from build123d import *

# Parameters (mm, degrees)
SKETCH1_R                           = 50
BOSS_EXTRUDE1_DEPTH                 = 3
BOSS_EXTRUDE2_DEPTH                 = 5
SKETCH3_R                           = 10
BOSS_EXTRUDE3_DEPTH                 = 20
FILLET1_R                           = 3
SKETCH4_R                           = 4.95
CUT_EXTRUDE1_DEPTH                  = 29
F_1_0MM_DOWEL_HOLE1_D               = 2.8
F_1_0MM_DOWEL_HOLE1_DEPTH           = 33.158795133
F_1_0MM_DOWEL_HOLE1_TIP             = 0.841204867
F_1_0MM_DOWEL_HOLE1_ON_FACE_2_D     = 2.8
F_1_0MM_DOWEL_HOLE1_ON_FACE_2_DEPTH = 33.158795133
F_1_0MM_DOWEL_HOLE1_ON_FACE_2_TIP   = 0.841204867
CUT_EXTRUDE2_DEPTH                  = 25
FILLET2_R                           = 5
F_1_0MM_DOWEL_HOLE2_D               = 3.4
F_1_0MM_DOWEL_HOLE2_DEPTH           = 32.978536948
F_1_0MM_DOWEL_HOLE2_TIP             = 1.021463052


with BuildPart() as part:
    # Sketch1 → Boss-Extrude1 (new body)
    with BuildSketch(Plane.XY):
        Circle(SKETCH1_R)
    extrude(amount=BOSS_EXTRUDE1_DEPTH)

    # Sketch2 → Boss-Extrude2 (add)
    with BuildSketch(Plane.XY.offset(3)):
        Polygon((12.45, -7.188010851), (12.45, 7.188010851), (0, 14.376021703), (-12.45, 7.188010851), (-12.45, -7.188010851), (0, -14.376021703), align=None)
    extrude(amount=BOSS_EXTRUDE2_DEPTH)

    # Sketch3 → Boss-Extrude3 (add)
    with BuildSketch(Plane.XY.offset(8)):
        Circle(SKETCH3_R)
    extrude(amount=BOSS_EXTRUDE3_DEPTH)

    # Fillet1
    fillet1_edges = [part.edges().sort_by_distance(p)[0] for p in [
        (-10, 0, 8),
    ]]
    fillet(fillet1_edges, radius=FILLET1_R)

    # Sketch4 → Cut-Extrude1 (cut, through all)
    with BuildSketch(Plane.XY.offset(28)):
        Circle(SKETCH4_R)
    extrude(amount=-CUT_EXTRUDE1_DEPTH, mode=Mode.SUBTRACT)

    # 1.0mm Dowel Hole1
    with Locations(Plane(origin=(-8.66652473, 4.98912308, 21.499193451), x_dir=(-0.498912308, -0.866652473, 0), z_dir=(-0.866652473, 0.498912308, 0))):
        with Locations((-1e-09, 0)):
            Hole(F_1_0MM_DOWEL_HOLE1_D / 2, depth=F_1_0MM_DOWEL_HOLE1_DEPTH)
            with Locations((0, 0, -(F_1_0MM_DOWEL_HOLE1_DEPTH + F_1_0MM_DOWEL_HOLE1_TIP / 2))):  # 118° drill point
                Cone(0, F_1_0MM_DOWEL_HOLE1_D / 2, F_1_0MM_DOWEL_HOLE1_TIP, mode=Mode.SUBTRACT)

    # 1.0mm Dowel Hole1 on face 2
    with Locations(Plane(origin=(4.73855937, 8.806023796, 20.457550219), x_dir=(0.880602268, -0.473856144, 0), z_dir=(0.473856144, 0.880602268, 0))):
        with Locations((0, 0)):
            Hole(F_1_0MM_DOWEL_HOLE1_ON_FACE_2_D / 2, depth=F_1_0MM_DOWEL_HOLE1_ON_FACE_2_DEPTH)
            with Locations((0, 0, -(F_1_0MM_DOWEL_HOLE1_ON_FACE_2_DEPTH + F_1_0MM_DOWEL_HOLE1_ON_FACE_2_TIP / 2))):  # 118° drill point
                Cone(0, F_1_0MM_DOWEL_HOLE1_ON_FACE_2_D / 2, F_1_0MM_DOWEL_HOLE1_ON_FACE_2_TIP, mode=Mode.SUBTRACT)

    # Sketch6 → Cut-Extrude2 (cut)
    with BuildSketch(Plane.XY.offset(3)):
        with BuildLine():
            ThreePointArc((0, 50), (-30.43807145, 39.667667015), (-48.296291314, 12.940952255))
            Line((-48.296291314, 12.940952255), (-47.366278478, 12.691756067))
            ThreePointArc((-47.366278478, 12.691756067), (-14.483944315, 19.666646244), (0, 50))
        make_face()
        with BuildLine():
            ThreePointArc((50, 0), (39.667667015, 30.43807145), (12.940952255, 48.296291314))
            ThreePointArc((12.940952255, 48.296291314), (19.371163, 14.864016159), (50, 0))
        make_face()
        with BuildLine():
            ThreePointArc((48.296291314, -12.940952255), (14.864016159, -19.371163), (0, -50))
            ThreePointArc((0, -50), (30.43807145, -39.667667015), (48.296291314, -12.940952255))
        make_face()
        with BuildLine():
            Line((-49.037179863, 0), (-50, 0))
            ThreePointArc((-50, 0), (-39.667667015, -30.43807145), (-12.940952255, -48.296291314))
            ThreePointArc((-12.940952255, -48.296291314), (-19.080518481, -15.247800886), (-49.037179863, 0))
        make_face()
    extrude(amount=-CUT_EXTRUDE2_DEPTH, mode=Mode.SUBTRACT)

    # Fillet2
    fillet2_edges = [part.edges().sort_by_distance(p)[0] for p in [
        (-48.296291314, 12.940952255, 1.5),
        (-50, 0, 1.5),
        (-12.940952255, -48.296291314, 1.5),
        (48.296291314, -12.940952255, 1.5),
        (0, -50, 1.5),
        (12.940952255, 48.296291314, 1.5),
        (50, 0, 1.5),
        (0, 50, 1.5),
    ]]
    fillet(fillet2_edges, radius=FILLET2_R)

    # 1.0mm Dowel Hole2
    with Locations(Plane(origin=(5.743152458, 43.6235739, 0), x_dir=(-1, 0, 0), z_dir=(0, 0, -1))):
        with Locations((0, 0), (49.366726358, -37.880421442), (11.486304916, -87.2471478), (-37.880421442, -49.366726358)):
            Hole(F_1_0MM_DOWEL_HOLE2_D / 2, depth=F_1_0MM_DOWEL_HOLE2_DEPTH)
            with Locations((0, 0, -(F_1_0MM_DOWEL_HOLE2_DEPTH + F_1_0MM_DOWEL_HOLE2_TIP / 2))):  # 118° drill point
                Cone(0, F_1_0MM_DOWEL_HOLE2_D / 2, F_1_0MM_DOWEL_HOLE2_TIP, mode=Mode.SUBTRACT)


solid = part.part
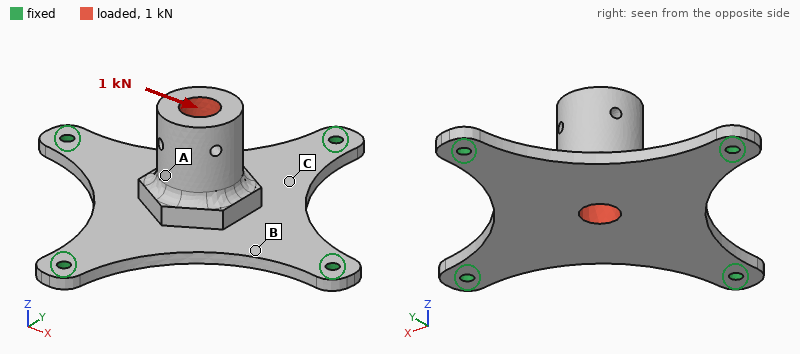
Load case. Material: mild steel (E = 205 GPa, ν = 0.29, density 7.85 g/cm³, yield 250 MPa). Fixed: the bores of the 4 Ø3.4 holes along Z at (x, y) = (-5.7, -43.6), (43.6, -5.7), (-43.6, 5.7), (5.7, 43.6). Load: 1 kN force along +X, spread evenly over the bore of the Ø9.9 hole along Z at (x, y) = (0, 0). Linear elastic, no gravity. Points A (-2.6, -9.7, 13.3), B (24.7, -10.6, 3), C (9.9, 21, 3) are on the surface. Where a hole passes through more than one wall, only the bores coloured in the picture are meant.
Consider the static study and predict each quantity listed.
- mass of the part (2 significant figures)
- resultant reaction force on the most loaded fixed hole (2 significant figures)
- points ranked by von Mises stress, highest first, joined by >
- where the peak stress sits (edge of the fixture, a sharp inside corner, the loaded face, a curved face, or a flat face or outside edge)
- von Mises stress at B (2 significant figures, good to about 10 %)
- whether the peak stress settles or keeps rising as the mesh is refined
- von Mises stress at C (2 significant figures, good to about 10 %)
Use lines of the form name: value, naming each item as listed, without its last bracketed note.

mass of the part: 140 g
resultant reaction force on the most loaded fixed hole: 470 N
points ranked by von Mises stress, highest first, joined by >: B > C > A
where the peak stress sits: edge of the fixture
von Mises stress at B: 46 MPa
whether the peak stress settles or keeps rising as the mesh is refined: keeps rising
von Mises stress at C: 13 MPa
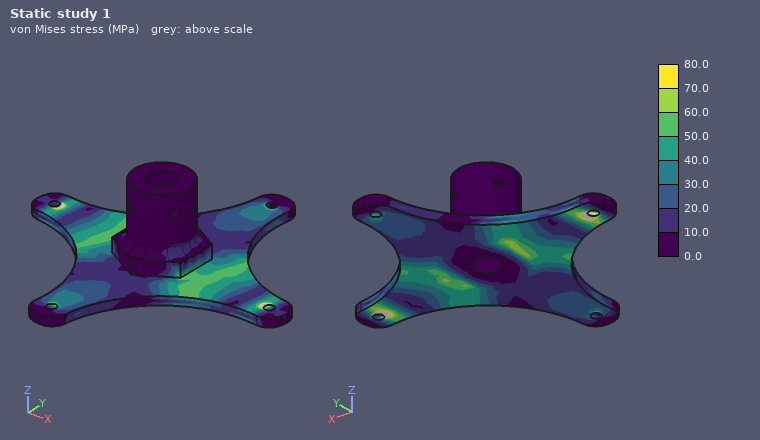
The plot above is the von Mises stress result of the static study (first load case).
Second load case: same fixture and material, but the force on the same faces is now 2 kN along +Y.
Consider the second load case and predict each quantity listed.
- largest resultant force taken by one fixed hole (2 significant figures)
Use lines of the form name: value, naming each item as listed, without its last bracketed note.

largest resultant force taken by one fixed hole: 940 N
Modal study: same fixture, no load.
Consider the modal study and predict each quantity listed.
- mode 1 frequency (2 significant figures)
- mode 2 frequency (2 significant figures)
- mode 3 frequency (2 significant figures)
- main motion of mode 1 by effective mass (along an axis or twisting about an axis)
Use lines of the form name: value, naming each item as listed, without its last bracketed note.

mode 1 frequency: 1800 Hz
mode 2 frequency: 3000 Hz
mode 3 frequency: 3000 Hz
main motion of mode 1 by effective mass: along Z
